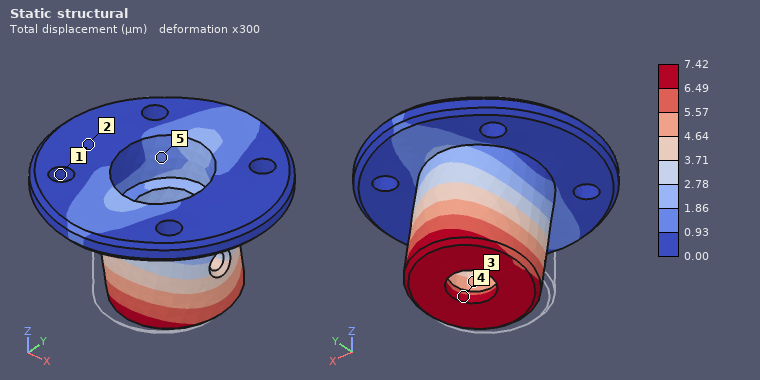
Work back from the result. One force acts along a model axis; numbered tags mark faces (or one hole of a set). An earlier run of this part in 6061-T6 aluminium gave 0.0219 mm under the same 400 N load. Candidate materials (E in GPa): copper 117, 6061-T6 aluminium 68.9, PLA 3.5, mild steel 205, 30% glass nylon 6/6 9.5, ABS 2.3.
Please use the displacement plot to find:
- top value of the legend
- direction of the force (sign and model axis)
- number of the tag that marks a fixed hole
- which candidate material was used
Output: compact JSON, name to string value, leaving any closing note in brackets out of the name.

{"top value of the legend": "7.42 µm", "direction of the force": "+Y", "number of the tag that marks a fixed hole": "1", "which candidate material was used": "mild steel"}
